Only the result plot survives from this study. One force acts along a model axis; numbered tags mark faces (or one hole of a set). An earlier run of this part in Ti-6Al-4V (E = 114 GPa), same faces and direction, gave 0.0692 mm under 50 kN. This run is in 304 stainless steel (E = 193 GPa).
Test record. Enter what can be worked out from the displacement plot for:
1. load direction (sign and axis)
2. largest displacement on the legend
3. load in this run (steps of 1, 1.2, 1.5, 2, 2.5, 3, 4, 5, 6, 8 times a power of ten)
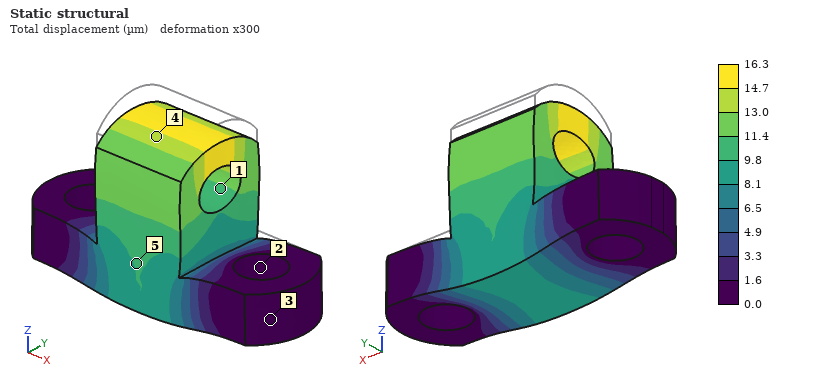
-Z
16.3 µm
20 kN
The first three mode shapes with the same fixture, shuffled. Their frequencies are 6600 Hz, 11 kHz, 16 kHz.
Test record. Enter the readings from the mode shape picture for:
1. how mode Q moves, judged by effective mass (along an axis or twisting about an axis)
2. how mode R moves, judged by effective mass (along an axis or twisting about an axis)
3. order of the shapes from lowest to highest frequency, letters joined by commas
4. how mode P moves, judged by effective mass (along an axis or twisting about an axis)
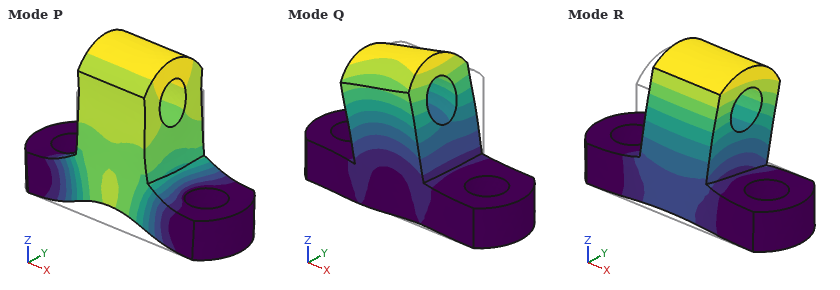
along X
along Y
R, Q, P
along Z
